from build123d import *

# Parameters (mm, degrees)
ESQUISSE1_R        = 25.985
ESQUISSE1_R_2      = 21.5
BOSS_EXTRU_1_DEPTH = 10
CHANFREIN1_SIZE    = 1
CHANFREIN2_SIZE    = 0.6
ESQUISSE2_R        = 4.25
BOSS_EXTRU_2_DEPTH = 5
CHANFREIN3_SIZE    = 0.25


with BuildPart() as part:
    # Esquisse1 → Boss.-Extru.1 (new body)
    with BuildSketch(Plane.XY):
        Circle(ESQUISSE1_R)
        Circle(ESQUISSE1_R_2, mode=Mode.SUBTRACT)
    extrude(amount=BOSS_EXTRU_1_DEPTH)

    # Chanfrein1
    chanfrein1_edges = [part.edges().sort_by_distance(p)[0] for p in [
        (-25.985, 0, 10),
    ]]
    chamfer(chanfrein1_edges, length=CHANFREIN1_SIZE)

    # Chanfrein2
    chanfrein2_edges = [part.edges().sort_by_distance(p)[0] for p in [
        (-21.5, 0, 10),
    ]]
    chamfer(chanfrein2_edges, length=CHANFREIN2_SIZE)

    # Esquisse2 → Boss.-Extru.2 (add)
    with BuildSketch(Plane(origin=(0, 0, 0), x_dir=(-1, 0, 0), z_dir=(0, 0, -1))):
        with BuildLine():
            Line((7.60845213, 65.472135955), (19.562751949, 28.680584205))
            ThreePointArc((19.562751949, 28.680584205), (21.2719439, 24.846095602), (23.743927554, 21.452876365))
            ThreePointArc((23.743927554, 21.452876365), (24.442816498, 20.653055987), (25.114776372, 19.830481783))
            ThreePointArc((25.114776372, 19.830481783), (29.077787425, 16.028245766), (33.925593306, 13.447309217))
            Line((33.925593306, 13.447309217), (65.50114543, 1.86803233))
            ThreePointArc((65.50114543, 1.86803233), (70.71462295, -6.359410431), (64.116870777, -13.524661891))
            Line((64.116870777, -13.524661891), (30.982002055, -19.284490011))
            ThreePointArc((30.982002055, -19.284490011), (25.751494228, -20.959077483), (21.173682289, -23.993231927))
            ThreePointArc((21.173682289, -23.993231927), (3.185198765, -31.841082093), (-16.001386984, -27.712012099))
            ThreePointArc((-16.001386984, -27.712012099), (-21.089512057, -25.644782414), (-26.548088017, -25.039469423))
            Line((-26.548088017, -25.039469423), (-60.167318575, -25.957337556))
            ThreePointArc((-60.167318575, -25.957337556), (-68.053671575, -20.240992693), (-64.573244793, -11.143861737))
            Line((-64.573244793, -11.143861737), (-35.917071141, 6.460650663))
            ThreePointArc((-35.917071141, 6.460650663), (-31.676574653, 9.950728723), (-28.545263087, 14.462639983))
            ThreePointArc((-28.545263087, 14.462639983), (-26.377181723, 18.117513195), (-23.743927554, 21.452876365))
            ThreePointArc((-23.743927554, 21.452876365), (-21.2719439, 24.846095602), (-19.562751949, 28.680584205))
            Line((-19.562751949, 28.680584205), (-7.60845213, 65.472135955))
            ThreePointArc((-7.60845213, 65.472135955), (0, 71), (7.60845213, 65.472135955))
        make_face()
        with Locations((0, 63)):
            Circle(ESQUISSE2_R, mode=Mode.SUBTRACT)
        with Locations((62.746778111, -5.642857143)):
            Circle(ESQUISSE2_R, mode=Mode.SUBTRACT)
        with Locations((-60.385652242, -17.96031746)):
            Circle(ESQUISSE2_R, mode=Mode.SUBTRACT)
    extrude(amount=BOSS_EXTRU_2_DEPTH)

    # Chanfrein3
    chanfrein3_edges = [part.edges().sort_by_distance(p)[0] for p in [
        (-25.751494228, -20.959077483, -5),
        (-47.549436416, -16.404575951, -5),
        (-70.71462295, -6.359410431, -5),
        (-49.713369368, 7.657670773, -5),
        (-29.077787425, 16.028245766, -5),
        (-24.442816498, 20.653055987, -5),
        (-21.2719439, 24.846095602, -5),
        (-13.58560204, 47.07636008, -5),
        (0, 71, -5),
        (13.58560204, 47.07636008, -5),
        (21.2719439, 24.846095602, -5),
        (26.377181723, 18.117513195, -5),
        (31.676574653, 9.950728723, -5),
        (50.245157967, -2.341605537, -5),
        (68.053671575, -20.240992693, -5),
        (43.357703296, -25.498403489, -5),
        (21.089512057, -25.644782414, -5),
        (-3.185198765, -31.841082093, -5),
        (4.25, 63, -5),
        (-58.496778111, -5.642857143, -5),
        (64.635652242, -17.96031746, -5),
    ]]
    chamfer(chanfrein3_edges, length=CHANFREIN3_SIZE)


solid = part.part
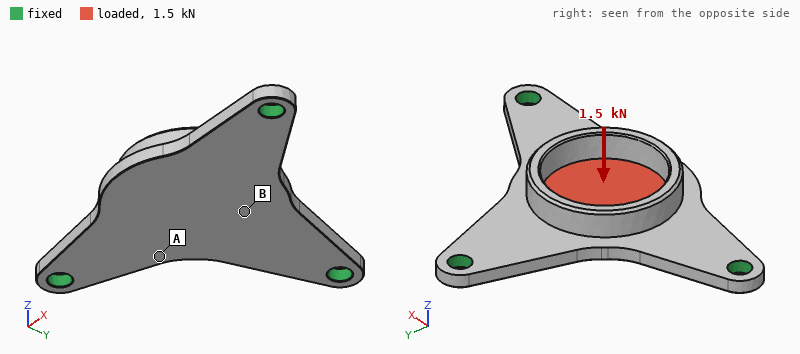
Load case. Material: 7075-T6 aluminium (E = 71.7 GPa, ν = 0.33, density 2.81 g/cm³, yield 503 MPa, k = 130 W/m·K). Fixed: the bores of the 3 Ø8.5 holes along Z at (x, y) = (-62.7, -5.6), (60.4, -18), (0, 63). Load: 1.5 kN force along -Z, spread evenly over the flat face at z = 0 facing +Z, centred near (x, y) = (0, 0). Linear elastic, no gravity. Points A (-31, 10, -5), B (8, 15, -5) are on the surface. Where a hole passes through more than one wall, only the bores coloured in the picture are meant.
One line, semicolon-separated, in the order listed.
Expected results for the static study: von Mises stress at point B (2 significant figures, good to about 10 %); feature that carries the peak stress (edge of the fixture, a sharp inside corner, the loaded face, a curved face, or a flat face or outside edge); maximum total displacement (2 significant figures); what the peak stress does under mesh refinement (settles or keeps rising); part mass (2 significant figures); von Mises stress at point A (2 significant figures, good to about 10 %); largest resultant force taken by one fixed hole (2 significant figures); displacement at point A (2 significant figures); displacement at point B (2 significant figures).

18 MPa; edge of the fixture; 0.27 mm; keeps rising; 100 g; 40 MPa; 650 N; 0.12 mm; 0.15 mm
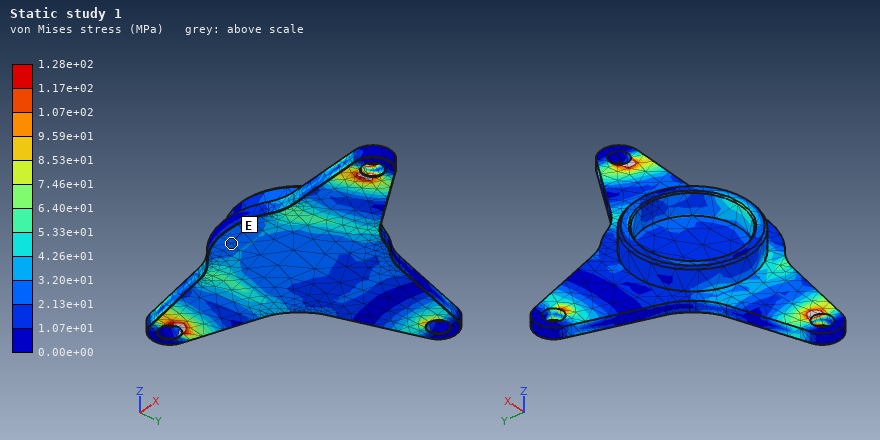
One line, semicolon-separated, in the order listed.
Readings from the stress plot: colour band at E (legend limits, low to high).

2.13e+01 to 3.20e+01 MPa
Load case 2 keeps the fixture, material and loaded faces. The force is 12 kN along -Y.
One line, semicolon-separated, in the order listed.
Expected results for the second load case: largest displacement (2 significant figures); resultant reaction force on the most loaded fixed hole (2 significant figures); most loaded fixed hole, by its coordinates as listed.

0.21 mm; 8.8 kN; (0, 63)
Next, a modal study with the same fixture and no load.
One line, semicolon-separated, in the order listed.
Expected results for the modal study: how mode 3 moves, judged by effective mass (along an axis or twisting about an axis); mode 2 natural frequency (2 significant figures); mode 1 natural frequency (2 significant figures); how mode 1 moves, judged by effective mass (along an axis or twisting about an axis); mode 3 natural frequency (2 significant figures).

twisting about Y; 3200 Hz; 1700 Hz; along Z; 4100 Hz
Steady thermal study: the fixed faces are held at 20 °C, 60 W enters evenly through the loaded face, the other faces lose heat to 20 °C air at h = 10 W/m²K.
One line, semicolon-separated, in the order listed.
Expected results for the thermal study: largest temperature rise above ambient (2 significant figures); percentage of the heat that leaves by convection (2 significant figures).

51 K; 8.0 %
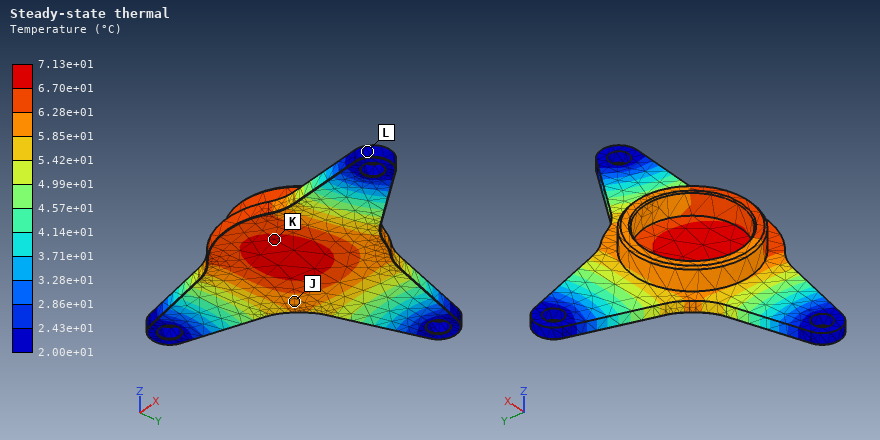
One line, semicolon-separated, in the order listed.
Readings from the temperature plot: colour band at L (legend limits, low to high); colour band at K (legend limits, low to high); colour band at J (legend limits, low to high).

2.00e+01 to 2.43e+01 °C; 6.70e+01 to 7.13e+01 °C; 5.85e+01 to 6.28e+01 °C
